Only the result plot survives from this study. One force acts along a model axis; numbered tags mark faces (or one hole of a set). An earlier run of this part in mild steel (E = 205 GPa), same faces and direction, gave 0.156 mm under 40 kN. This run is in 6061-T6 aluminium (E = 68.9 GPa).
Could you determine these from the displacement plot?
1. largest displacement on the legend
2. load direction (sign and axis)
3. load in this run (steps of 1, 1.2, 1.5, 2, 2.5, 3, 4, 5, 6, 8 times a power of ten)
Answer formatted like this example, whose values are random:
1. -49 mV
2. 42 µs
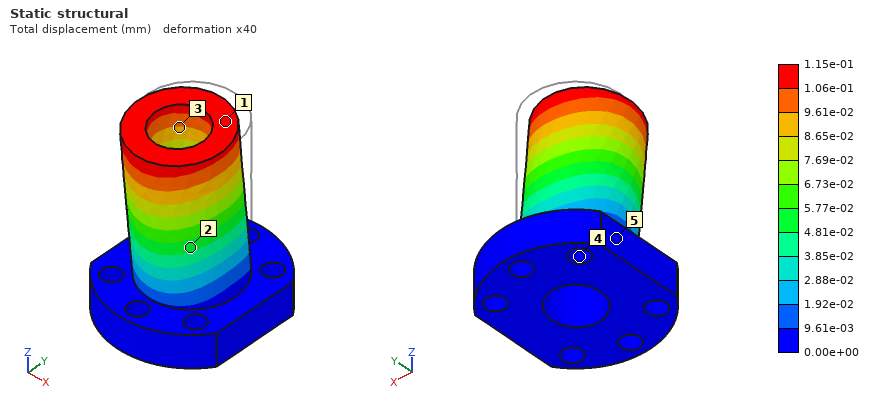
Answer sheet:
1. 1.15e-01 mm
2. -Y
3. 10 kN
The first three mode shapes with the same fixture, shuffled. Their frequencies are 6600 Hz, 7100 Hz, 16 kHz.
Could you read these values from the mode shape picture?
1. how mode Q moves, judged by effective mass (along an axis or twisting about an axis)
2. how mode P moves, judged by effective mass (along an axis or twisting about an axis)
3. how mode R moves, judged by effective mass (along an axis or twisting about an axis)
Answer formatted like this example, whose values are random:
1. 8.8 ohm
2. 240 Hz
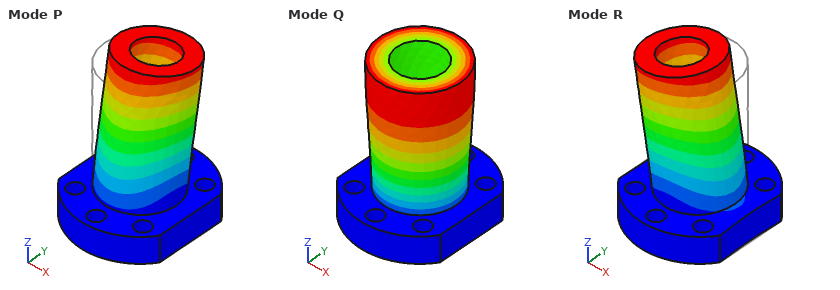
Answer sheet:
1. twisting about Z
2. along Y
3. along X
